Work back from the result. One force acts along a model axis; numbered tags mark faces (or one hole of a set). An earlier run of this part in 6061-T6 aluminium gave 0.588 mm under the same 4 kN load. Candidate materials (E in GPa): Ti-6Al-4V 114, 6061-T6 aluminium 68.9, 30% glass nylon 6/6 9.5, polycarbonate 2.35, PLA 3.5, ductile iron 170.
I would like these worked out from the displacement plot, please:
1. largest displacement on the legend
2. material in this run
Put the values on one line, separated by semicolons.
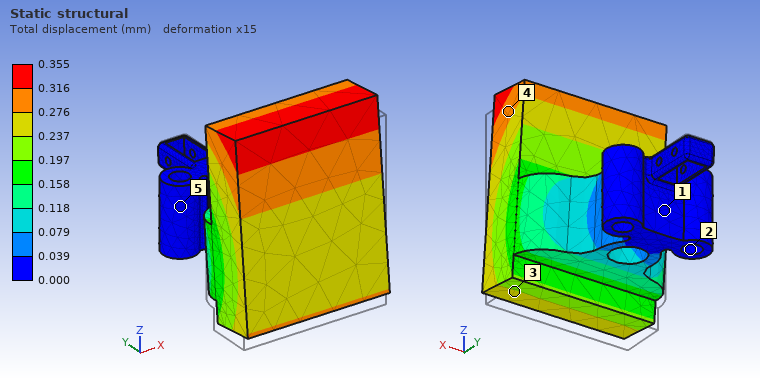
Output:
0.355 mm; Ti-6Al-4V
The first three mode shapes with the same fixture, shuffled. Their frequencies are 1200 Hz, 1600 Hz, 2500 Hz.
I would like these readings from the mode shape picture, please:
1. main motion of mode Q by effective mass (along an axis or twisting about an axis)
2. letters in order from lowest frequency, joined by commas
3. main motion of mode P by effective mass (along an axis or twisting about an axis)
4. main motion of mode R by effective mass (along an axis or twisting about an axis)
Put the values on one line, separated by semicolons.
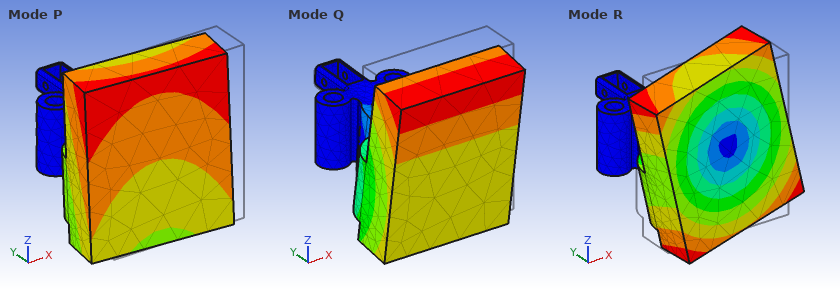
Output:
along Z; P, Q, R; along X; twisting about Y
